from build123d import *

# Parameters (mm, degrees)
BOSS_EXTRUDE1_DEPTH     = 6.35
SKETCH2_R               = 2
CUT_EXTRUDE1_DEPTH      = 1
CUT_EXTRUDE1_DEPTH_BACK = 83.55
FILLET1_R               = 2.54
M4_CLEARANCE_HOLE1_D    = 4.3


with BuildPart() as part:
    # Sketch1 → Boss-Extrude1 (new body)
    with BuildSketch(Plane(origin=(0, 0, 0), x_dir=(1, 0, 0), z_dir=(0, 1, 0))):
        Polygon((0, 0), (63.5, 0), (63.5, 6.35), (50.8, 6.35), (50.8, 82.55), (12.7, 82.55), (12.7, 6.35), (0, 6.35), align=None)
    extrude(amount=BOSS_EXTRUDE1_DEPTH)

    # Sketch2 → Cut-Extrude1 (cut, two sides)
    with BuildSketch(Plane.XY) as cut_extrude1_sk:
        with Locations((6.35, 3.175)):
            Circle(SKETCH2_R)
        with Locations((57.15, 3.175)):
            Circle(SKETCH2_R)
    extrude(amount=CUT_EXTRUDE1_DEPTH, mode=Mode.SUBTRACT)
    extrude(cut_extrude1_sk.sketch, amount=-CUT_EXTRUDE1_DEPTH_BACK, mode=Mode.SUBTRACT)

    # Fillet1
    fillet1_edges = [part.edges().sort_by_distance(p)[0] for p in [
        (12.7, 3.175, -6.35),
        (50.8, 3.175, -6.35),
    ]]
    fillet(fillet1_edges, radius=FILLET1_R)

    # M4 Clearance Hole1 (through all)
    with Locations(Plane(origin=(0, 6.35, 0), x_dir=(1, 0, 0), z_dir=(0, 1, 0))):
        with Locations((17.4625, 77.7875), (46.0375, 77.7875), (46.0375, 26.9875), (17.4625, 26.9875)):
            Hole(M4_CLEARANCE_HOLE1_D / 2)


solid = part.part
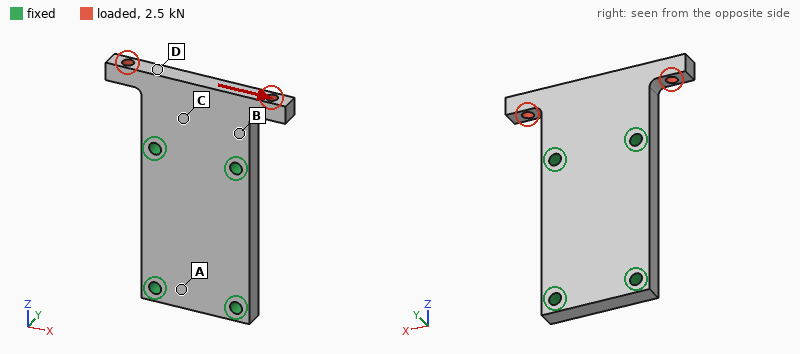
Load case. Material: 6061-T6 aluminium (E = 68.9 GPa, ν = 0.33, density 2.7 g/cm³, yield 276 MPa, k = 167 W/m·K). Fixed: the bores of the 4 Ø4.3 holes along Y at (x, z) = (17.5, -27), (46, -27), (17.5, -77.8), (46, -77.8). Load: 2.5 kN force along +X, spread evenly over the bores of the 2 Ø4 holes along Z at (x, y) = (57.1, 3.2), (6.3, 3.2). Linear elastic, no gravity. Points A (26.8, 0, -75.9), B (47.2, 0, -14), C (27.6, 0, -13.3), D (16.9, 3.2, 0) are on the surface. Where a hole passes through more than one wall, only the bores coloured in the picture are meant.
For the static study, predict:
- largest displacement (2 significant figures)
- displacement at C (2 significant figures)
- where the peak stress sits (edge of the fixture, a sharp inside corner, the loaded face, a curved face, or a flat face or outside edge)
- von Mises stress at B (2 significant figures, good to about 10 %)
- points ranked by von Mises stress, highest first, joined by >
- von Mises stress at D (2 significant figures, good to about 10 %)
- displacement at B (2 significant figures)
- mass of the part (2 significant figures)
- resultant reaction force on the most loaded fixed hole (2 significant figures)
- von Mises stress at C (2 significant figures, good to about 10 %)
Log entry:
37 µm
8.5 µm
the loaded face
16 MPa
D > C > B > A
38 MPa
9.4 µm
55 g
2.3 kN
27 MPa
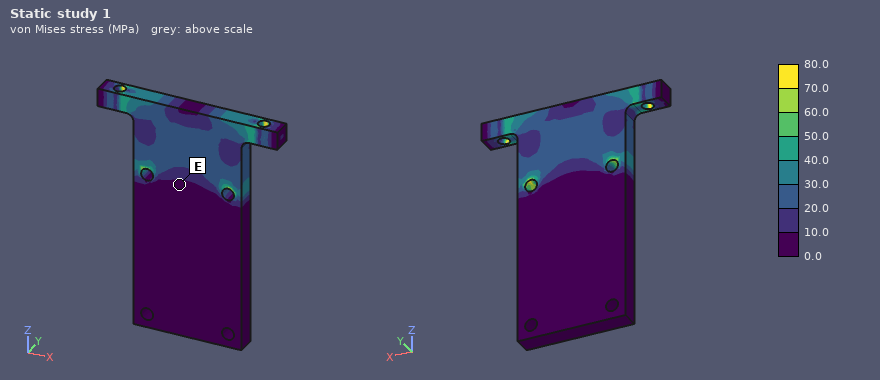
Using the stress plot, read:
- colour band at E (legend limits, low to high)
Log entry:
0.0 to 10.0 MPa
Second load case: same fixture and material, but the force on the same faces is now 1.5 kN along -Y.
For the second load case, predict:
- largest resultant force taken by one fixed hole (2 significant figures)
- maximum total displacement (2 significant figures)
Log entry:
800 N
0.30 mm
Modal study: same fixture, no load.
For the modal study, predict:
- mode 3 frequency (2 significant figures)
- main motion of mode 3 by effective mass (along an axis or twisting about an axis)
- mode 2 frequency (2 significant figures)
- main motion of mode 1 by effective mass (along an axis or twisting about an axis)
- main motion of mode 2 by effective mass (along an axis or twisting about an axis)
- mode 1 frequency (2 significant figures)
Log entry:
11 kHz
along Y
7300 Hz
along Y
twisting about Z
5600 Hz
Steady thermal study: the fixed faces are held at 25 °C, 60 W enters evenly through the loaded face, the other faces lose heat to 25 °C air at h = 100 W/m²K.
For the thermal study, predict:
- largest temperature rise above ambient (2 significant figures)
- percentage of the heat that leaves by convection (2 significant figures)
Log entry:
85 K
17 %
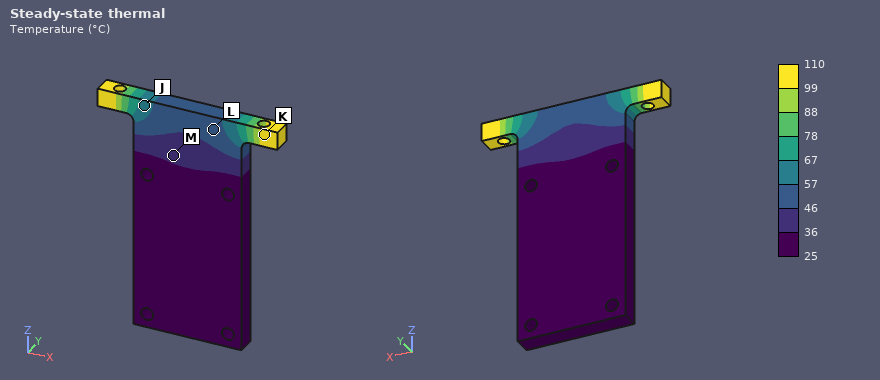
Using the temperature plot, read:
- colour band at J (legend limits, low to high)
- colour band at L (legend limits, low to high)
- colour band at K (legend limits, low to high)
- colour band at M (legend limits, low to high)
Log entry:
57 to 67 °C
46 to 57 °C
99 to 110 °C
36 to 46 °C
